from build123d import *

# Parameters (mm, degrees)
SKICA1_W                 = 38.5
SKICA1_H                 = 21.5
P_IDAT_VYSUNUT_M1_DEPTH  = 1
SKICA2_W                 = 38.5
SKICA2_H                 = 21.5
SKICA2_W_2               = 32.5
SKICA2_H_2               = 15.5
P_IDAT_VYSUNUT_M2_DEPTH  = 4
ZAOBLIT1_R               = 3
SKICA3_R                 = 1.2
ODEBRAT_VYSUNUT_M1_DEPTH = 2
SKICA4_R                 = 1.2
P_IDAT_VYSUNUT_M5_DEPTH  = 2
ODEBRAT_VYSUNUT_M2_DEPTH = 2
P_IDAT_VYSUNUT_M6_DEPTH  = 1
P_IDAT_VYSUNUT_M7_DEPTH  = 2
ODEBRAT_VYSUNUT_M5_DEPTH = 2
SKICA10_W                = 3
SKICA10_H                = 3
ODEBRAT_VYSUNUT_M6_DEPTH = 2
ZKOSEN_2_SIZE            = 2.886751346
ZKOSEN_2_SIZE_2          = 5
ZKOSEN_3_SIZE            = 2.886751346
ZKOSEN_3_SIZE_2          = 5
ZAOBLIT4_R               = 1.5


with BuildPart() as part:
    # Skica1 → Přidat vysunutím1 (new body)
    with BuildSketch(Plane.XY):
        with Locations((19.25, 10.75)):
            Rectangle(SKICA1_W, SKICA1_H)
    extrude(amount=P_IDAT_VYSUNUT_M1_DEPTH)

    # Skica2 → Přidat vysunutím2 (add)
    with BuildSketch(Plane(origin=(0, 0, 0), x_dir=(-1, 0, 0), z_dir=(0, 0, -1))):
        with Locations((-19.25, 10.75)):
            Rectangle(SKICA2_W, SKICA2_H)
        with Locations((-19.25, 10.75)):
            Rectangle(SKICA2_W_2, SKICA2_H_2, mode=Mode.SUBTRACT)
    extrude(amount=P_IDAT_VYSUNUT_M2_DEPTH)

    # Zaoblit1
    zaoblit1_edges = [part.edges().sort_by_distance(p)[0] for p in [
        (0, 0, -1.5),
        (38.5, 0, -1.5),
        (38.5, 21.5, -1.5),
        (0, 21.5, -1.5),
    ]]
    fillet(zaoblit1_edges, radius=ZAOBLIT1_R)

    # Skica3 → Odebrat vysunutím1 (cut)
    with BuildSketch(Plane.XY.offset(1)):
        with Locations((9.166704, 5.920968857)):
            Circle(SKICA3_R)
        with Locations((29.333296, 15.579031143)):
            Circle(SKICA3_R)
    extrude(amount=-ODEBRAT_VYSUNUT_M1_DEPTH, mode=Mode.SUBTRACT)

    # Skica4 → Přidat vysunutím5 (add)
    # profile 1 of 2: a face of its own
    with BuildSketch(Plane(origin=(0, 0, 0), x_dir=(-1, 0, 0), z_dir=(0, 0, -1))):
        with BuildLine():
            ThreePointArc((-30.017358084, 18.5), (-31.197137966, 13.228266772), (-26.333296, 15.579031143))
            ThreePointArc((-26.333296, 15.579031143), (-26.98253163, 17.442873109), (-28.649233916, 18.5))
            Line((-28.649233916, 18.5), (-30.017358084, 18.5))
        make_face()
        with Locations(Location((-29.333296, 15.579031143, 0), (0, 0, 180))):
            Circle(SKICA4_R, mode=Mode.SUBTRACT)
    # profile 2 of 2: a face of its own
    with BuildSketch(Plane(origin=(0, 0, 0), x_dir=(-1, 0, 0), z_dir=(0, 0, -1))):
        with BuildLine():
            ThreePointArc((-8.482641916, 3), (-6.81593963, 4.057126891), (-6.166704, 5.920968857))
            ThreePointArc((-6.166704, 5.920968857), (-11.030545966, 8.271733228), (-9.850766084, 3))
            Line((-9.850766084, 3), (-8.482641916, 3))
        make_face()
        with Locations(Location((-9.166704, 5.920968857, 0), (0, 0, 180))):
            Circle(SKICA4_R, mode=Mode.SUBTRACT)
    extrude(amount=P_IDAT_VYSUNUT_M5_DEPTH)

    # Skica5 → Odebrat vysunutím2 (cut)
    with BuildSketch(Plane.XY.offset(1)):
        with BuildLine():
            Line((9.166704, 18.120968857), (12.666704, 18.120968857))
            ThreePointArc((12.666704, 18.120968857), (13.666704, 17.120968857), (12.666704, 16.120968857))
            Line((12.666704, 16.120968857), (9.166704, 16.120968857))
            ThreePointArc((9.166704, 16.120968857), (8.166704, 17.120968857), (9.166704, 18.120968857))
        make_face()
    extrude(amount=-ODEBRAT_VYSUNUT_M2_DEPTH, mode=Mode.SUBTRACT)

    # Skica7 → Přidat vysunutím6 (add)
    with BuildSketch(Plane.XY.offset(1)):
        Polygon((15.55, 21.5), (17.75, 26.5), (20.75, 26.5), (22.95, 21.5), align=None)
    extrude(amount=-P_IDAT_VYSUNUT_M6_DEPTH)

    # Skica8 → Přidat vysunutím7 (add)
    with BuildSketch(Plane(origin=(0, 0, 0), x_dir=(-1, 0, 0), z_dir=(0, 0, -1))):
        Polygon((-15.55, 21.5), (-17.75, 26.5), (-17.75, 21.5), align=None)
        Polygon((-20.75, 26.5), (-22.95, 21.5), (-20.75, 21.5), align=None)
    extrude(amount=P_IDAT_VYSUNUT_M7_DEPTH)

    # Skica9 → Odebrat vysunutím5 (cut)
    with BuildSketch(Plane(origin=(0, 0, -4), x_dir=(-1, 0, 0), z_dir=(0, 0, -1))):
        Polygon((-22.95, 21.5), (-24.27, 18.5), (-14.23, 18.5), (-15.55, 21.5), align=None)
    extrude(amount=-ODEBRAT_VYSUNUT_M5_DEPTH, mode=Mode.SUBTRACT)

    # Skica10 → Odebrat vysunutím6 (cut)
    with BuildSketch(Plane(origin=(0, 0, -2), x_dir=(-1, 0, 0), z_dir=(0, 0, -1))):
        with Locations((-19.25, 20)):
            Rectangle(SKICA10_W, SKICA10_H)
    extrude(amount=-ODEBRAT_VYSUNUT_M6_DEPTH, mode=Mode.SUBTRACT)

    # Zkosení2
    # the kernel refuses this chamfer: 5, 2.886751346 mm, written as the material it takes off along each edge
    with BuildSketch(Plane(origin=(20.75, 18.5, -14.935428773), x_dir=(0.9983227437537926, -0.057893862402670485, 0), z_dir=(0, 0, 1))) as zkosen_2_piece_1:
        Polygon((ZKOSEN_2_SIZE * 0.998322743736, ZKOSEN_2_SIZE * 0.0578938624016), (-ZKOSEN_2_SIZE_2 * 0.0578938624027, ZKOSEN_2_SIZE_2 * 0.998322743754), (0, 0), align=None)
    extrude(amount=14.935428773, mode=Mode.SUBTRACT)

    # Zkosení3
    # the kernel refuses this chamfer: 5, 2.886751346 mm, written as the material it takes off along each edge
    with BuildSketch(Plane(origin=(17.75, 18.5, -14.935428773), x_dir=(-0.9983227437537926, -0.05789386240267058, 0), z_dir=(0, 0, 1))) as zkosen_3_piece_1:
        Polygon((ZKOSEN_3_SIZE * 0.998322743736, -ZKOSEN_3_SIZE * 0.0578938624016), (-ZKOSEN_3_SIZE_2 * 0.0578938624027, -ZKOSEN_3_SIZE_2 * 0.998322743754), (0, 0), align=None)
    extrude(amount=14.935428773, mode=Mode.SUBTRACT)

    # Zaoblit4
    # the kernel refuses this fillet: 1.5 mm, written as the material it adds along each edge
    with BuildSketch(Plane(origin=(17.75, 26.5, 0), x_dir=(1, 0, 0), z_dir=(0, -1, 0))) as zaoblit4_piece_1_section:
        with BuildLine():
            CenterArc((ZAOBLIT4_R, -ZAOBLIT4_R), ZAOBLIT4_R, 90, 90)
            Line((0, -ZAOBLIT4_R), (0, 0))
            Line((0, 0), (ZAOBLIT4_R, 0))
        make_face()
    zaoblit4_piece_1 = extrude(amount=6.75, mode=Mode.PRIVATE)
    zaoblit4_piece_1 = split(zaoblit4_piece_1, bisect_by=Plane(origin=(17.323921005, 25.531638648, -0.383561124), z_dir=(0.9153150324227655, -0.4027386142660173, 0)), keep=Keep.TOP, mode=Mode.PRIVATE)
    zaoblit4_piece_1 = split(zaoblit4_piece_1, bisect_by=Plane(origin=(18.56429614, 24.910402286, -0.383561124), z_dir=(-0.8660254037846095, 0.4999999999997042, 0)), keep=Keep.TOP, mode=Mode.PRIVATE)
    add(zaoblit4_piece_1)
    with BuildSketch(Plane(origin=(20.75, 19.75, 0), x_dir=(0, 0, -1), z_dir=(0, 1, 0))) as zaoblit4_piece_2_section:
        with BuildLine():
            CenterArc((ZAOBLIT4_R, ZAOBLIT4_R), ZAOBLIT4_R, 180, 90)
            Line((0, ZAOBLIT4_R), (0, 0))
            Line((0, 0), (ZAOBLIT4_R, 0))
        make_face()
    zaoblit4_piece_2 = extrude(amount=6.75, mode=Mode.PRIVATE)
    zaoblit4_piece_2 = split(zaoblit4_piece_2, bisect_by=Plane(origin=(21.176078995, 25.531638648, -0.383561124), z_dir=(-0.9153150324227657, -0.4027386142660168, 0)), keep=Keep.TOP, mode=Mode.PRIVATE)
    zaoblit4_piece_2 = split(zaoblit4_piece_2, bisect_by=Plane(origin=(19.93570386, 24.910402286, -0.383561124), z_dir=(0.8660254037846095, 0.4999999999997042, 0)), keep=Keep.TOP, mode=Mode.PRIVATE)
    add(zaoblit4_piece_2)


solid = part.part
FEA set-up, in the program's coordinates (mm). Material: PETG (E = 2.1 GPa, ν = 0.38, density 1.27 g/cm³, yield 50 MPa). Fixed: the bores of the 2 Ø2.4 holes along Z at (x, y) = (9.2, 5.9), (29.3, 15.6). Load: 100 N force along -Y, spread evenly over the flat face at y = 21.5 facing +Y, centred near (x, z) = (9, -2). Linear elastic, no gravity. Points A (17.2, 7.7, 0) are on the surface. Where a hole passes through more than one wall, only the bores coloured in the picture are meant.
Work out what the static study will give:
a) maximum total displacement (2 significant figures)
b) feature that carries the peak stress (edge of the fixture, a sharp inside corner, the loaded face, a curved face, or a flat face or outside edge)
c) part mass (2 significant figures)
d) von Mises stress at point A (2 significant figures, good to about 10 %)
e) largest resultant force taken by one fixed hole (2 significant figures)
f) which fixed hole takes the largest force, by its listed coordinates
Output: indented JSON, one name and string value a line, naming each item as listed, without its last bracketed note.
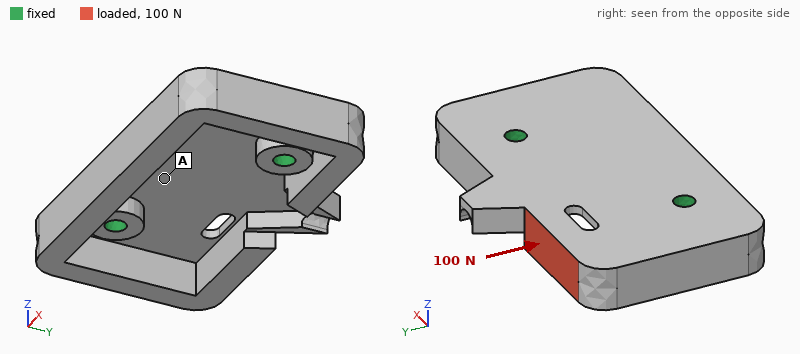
{
  "maximum total displacement": "0.53 mm",
  "feature that carries the peak stress": "a curved face",
  "part mass": "2.7 g",
  "von Mises stress at point A": "2.5 MPa",
  "largest resultant force taken by one fixed hole": "94 N",
  "which fixed hole takes the largest force, by its listed coordinates": "(9.2, 5.9)"
}
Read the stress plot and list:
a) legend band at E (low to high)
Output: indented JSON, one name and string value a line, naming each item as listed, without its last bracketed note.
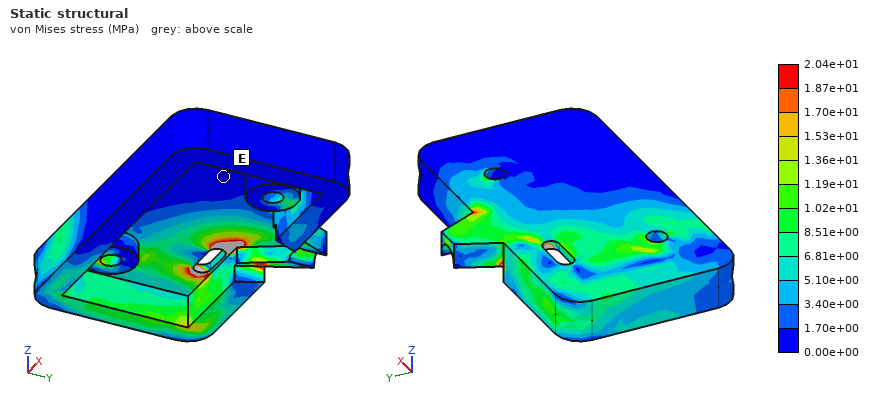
{
  "legend band at E": "0.00e+00 to 1.70e+00 MPa"
}
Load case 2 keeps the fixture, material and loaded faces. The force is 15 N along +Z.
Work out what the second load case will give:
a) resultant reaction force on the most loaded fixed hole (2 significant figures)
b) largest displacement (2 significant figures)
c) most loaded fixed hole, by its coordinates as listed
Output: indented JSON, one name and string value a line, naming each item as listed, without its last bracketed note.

{
  "resultant reaction force on the most loaded fixed hole": "11 N",
  "largest displacement": "0.52 mm",
  "most loaded fixed hole, by its coordinates as listed": "(9.2, 5.9)"
}
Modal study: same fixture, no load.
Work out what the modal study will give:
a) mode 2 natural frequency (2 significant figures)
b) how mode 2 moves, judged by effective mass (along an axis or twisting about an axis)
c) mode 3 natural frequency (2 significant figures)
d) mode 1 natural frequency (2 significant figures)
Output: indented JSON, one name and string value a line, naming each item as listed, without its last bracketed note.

{
  "mode 2 natural frequency": "1700 Hz",
  "how mode 2 moves, judged by effective mass": "along Z",
  "mode 3 natural frequency": "2800 Hz",
  "mode 1 natural frequency": "1300 Hz"
}
